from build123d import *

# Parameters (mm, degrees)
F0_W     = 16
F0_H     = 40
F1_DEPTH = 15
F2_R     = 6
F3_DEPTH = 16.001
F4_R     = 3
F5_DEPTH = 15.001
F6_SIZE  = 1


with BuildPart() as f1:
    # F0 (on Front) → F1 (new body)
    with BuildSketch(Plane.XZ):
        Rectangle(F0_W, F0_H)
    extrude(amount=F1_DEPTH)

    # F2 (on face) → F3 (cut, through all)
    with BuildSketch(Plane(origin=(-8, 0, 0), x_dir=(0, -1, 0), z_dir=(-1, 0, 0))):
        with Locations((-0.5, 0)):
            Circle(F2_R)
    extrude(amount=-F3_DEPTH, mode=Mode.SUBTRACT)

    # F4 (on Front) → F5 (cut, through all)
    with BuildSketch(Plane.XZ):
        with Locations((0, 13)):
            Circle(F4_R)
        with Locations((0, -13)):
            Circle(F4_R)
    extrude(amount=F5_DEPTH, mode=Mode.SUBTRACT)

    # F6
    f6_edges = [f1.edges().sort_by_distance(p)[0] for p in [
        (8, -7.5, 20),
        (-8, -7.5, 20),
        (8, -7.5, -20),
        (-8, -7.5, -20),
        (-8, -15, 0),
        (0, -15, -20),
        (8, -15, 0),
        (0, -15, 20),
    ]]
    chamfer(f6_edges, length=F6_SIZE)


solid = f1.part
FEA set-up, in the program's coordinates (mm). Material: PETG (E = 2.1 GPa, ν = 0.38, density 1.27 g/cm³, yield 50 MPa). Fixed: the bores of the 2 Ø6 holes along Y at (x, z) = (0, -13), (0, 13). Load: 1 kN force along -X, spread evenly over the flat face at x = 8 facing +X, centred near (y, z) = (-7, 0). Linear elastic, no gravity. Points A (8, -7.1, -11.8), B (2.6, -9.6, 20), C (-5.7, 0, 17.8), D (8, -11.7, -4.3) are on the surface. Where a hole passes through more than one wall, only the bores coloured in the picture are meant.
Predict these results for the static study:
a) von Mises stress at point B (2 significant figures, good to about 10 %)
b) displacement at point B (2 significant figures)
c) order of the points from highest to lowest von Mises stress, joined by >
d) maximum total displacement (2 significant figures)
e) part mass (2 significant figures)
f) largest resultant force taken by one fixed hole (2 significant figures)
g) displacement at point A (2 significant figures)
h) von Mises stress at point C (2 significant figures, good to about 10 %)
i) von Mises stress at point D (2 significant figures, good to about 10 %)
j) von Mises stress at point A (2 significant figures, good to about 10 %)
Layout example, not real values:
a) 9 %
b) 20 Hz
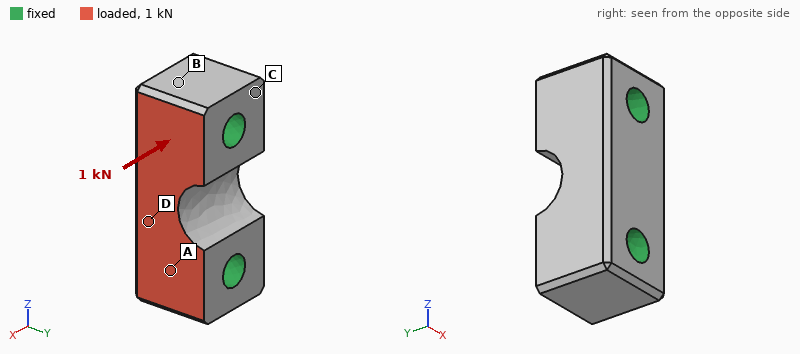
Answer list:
a) 0.81 MPa
b) 3.0 µm
c) A > D > B > C
d) 18 µm
e) 10.0 g
f) 500 N
g) 6.8 µm
h) 0.52 MPa
i) 1.6 MPa
j) 2.9 MPa
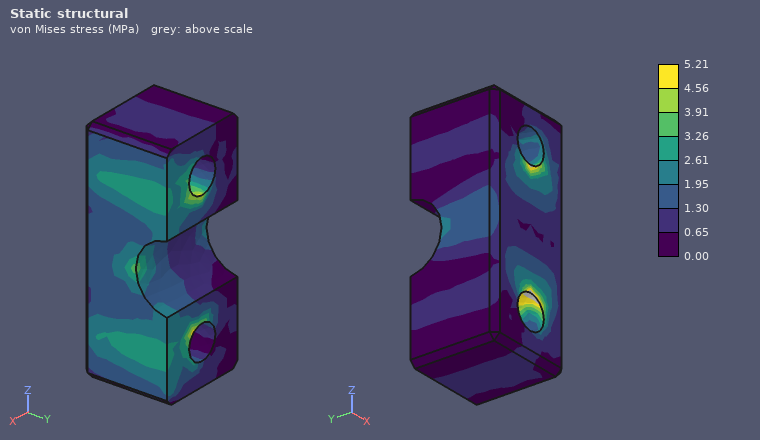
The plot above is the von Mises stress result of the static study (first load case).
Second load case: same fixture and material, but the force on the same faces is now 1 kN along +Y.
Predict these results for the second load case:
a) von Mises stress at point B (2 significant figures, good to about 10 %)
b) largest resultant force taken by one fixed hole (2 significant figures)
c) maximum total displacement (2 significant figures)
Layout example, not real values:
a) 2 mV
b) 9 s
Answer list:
a) 1.3 MPa
b) 500 N
c) 51 µm
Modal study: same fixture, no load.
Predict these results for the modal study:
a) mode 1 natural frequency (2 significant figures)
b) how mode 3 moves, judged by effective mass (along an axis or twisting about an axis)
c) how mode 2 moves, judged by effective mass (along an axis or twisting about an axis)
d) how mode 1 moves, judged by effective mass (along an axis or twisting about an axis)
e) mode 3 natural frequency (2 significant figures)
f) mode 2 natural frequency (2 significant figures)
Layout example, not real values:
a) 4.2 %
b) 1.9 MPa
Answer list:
a) 14 kHz
b) twisting about Z
c) along Y
d) along X
e) 18 kHz
f) 15 kHz
